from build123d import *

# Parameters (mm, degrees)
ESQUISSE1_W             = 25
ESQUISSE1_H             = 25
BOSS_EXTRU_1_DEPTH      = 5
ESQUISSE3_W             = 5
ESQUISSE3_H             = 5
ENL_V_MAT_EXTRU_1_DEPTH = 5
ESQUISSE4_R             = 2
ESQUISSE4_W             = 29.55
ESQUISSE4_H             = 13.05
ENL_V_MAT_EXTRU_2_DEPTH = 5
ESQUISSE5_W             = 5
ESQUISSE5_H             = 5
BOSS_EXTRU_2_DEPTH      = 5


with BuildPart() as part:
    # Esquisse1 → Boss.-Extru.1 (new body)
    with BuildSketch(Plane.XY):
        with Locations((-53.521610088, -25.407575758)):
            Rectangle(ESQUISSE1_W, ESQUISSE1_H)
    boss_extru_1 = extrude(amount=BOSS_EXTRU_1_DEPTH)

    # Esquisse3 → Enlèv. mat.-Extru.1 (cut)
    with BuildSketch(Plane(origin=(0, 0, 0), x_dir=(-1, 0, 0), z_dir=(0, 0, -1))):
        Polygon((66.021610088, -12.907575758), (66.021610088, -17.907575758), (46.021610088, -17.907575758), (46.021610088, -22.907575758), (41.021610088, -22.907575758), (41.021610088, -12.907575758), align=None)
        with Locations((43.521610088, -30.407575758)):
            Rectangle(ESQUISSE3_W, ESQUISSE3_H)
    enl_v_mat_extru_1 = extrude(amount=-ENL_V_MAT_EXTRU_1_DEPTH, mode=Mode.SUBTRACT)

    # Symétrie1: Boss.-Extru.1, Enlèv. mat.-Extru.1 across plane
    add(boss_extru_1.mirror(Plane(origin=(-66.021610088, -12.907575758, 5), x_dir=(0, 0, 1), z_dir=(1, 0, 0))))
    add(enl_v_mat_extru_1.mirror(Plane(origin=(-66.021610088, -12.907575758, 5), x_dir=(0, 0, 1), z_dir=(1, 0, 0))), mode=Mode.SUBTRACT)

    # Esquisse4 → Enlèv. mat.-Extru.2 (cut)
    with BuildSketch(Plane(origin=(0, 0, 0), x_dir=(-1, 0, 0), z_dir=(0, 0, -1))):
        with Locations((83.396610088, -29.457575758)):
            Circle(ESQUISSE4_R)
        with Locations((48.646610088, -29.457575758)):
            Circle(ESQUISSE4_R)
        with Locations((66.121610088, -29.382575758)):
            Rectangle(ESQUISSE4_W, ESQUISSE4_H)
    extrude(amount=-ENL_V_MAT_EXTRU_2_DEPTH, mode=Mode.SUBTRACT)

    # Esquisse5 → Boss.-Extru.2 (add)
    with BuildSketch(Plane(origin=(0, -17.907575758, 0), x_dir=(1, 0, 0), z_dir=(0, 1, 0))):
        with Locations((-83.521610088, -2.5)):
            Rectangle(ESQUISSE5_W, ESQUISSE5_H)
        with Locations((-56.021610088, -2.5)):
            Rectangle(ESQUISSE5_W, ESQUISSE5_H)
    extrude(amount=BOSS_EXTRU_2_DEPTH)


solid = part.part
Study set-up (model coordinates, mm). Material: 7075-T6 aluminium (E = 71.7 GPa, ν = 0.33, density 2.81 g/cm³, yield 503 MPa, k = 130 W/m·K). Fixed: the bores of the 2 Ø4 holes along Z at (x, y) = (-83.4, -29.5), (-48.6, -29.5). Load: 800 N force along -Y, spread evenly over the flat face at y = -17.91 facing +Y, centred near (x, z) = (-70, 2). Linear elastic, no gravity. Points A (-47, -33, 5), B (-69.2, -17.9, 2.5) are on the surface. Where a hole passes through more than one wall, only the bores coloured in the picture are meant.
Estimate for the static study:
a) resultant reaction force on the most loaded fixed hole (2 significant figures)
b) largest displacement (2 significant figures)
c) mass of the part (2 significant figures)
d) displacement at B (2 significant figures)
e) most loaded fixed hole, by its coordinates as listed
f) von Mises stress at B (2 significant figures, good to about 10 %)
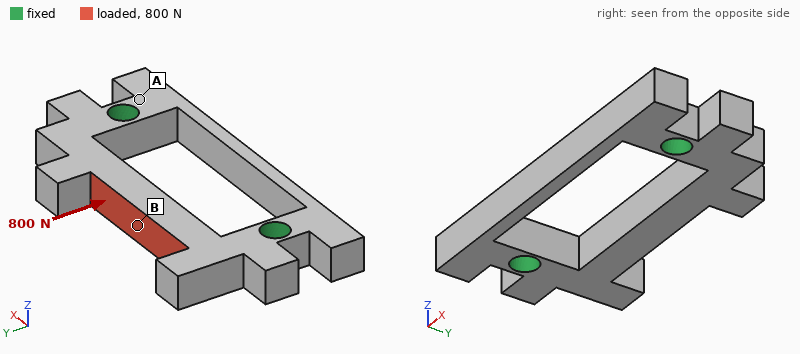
610 N
46 µm
7.6 g
43 µm
(-83.4, -29.5)
94 MPa
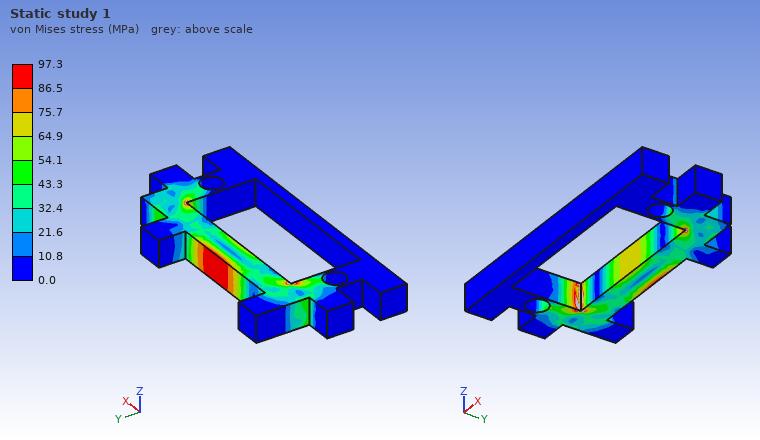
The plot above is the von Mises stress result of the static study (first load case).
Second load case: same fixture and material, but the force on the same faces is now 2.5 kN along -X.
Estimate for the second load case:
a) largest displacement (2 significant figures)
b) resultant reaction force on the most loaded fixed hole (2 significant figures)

67 µm
1.3 kN
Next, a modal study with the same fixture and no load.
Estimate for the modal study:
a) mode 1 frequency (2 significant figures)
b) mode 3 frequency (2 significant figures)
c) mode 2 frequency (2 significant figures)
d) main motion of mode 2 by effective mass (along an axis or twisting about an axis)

10000 Hz
16 kHz
11 kHz
along Z
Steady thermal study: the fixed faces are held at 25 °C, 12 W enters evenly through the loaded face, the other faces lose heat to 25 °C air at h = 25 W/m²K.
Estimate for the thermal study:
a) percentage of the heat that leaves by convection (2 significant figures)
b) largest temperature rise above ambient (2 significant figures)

3.5 %
29 K
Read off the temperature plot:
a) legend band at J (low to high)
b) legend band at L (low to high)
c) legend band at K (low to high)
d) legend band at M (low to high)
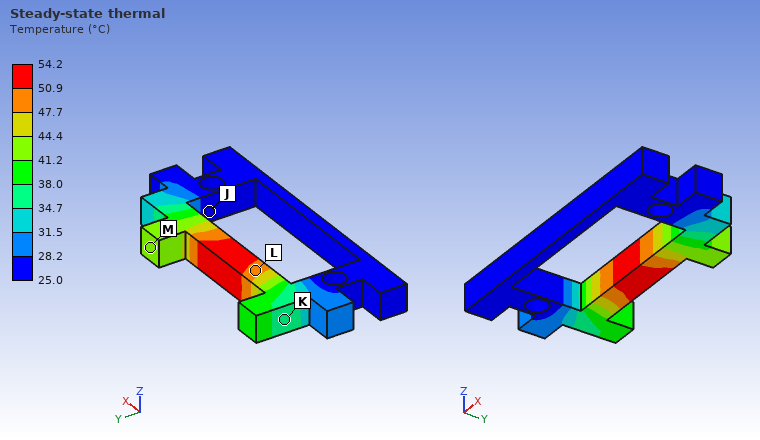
25.0 to 28.2 °C
47.7 to 50.9 °C
34.7 to 38.0 °C
41.2 to 44.4 °C
